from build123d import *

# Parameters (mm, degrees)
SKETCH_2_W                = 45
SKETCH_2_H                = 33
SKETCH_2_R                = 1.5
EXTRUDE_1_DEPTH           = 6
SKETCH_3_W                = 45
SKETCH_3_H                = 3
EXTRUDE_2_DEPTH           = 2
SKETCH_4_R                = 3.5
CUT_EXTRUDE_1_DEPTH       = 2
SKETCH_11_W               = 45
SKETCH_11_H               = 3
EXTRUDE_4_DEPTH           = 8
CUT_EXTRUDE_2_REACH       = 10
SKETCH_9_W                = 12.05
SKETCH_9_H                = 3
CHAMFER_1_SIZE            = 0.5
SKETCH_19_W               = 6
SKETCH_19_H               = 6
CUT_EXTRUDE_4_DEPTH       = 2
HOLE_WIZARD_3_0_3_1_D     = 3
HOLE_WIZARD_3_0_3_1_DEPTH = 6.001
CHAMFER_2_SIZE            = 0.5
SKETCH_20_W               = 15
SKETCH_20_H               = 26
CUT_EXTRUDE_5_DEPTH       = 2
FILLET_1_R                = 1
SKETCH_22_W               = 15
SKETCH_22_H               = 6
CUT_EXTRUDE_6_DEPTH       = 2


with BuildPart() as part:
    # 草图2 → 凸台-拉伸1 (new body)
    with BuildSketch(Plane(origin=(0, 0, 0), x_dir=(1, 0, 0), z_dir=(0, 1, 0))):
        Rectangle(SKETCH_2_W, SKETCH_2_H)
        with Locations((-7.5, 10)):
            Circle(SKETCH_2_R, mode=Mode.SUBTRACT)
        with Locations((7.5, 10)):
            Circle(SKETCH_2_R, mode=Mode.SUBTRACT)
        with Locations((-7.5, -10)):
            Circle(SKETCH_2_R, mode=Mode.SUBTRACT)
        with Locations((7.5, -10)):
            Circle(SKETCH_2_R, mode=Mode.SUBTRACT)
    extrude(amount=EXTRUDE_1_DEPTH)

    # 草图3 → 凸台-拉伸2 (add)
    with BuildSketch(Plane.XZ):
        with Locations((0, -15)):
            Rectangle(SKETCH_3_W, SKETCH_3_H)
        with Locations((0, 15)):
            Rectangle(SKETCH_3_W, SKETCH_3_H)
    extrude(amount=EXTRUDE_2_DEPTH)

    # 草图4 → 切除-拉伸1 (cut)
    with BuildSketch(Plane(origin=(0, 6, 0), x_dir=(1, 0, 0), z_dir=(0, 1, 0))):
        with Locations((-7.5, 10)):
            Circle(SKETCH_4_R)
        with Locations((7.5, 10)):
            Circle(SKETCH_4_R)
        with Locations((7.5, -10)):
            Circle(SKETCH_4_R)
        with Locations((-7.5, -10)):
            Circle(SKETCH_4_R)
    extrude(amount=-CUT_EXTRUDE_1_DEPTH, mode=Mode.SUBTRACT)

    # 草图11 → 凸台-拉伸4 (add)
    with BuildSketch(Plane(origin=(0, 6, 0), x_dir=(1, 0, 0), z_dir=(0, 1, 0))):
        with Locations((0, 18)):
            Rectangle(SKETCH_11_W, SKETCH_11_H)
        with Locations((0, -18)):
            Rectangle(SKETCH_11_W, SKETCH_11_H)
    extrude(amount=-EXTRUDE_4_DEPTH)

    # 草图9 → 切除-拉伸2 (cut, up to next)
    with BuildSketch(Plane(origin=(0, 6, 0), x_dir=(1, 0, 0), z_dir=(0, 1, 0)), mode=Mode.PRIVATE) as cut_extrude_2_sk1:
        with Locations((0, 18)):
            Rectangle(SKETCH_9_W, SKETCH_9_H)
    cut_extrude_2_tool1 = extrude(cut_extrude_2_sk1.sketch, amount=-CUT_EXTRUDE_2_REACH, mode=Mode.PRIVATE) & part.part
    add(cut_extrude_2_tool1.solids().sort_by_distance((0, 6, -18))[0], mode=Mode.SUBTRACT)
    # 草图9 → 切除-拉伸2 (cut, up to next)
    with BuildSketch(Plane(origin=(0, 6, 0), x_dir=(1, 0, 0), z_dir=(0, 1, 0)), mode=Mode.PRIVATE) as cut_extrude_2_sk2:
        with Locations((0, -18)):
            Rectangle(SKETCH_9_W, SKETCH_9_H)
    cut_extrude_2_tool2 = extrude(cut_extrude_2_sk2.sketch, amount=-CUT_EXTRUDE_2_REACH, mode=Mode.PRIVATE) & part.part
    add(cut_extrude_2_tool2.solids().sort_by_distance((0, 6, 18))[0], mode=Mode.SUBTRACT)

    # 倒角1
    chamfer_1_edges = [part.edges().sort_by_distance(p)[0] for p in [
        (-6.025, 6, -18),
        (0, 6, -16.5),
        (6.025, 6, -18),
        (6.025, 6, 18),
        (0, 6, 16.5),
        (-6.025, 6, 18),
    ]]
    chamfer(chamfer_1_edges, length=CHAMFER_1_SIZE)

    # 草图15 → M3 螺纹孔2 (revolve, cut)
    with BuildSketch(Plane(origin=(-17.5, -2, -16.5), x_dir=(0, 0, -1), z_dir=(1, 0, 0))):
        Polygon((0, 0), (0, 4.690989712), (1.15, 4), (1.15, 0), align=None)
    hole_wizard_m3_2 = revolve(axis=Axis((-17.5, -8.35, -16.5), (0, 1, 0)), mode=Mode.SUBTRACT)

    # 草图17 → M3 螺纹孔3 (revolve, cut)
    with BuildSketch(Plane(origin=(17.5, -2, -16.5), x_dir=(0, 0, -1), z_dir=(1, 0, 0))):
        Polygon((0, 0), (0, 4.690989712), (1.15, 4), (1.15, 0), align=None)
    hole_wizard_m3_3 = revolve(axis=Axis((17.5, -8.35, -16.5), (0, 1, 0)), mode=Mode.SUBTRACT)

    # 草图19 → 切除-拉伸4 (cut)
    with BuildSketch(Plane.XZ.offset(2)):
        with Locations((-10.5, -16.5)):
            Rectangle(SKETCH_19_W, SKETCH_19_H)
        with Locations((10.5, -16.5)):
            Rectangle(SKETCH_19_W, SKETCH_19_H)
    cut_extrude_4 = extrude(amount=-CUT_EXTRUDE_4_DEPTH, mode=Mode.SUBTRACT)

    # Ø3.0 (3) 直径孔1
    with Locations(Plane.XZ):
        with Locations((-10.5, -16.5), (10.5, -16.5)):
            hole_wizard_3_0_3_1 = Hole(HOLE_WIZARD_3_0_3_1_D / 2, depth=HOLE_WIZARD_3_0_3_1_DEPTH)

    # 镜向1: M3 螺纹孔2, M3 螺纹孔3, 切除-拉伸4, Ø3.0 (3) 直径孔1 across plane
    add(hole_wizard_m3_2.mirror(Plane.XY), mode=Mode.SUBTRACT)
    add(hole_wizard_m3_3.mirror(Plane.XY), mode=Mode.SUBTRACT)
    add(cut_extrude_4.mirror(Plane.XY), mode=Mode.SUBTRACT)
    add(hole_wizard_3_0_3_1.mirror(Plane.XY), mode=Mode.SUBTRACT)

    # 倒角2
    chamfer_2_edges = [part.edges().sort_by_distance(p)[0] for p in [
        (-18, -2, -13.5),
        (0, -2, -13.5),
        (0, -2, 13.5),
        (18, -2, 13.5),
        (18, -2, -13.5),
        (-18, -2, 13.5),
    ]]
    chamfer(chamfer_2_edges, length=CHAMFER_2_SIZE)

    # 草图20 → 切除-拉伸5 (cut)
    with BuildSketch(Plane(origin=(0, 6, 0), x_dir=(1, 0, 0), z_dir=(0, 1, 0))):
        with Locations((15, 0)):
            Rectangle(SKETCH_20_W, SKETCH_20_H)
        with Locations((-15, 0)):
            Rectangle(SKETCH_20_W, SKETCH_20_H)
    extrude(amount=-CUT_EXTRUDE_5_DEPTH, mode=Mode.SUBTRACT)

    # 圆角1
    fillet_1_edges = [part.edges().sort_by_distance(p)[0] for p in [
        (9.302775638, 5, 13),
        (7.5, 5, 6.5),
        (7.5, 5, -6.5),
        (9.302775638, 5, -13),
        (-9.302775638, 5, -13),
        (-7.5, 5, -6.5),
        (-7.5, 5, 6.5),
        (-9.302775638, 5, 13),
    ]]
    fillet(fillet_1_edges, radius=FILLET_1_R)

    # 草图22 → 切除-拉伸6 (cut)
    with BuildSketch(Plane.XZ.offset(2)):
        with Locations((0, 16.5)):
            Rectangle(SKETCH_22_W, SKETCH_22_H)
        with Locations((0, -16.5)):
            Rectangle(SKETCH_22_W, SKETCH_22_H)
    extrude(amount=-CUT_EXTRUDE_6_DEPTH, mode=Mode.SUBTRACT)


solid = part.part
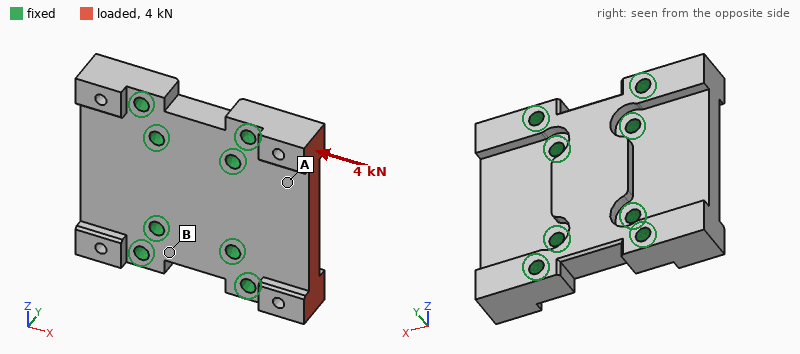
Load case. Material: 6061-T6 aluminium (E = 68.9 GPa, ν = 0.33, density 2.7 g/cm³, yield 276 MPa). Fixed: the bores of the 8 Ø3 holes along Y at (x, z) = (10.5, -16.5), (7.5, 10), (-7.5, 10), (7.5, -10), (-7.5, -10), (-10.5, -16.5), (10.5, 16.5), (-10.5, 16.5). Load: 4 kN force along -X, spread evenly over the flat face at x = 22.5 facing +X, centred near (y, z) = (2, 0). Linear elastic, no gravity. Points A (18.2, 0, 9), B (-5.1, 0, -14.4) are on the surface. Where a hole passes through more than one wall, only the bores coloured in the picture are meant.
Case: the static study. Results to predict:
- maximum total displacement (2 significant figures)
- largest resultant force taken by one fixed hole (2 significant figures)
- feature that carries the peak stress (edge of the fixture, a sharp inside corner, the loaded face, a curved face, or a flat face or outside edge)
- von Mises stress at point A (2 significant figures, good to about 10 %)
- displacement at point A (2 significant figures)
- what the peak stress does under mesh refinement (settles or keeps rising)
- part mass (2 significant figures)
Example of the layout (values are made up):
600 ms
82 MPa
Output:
8.0 µm
1.1 kN
edge of the fixture
20 MPa
4.4 µm
keeps rising
23 g
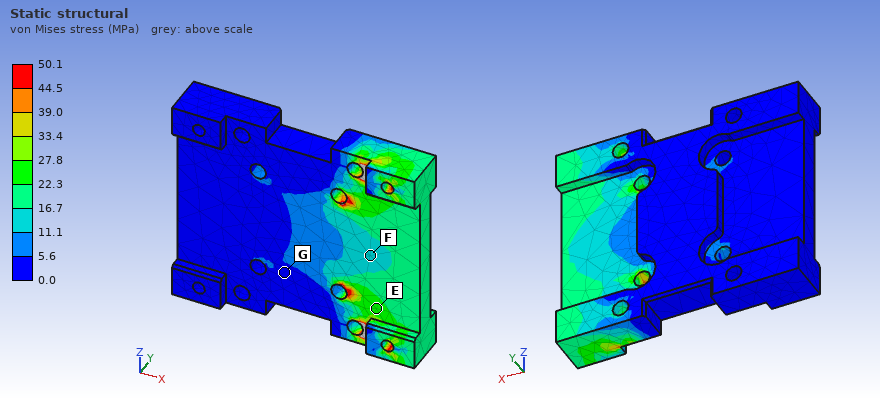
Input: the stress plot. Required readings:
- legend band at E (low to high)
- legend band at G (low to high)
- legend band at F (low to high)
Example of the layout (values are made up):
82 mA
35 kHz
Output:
22.3 to 27.8 MPa
0.0 to 5.6 MPa
11.1 to 16.7 MPa
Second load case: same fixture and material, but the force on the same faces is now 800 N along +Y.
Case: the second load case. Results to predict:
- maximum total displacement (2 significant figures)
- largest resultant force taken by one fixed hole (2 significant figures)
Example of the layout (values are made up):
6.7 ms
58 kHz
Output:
31 µm
360 N
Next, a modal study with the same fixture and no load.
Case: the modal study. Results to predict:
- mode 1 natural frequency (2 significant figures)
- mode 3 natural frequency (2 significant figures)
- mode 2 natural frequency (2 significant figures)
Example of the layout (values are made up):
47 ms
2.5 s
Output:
20 kHz
28 kHz
20 kHz
